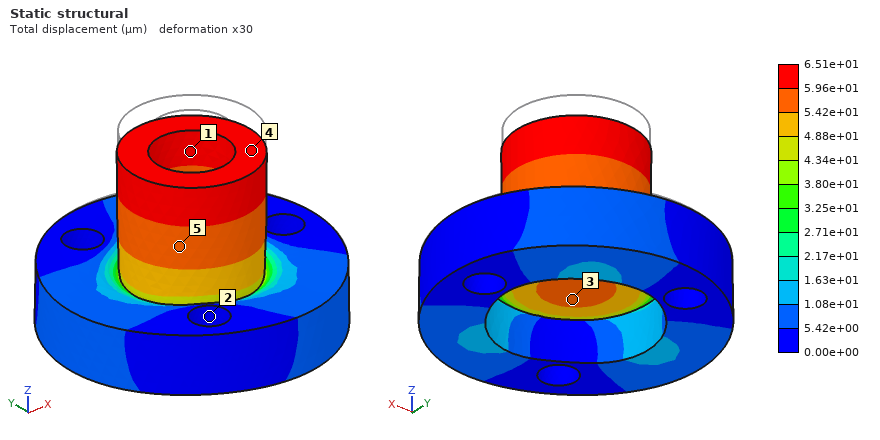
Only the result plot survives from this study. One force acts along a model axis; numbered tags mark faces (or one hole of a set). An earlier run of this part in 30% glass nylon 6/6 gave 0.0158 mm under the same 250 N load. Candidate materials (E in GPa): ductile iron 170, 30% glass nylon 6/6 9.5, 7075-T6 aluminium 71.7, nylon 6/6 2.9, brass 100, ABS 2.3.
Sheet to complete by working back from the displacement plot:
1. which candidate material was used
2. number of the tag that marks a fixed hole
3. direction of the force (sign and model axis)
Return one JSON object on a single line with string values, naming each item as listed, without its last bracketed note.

{"which candidate material was used": "ABS", "number of the tag that marks a fixed hole": "2", "direction of the force": "-Z"}
